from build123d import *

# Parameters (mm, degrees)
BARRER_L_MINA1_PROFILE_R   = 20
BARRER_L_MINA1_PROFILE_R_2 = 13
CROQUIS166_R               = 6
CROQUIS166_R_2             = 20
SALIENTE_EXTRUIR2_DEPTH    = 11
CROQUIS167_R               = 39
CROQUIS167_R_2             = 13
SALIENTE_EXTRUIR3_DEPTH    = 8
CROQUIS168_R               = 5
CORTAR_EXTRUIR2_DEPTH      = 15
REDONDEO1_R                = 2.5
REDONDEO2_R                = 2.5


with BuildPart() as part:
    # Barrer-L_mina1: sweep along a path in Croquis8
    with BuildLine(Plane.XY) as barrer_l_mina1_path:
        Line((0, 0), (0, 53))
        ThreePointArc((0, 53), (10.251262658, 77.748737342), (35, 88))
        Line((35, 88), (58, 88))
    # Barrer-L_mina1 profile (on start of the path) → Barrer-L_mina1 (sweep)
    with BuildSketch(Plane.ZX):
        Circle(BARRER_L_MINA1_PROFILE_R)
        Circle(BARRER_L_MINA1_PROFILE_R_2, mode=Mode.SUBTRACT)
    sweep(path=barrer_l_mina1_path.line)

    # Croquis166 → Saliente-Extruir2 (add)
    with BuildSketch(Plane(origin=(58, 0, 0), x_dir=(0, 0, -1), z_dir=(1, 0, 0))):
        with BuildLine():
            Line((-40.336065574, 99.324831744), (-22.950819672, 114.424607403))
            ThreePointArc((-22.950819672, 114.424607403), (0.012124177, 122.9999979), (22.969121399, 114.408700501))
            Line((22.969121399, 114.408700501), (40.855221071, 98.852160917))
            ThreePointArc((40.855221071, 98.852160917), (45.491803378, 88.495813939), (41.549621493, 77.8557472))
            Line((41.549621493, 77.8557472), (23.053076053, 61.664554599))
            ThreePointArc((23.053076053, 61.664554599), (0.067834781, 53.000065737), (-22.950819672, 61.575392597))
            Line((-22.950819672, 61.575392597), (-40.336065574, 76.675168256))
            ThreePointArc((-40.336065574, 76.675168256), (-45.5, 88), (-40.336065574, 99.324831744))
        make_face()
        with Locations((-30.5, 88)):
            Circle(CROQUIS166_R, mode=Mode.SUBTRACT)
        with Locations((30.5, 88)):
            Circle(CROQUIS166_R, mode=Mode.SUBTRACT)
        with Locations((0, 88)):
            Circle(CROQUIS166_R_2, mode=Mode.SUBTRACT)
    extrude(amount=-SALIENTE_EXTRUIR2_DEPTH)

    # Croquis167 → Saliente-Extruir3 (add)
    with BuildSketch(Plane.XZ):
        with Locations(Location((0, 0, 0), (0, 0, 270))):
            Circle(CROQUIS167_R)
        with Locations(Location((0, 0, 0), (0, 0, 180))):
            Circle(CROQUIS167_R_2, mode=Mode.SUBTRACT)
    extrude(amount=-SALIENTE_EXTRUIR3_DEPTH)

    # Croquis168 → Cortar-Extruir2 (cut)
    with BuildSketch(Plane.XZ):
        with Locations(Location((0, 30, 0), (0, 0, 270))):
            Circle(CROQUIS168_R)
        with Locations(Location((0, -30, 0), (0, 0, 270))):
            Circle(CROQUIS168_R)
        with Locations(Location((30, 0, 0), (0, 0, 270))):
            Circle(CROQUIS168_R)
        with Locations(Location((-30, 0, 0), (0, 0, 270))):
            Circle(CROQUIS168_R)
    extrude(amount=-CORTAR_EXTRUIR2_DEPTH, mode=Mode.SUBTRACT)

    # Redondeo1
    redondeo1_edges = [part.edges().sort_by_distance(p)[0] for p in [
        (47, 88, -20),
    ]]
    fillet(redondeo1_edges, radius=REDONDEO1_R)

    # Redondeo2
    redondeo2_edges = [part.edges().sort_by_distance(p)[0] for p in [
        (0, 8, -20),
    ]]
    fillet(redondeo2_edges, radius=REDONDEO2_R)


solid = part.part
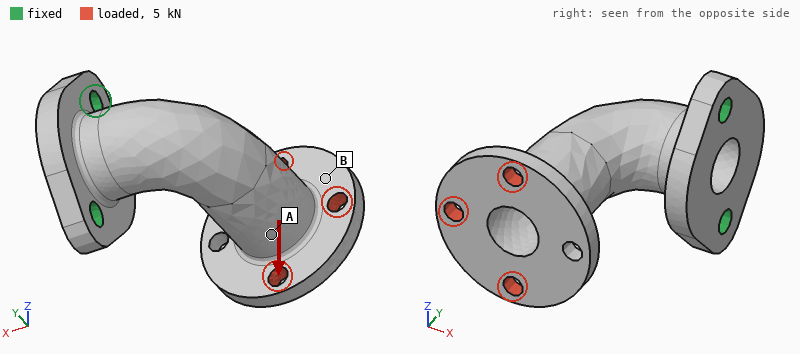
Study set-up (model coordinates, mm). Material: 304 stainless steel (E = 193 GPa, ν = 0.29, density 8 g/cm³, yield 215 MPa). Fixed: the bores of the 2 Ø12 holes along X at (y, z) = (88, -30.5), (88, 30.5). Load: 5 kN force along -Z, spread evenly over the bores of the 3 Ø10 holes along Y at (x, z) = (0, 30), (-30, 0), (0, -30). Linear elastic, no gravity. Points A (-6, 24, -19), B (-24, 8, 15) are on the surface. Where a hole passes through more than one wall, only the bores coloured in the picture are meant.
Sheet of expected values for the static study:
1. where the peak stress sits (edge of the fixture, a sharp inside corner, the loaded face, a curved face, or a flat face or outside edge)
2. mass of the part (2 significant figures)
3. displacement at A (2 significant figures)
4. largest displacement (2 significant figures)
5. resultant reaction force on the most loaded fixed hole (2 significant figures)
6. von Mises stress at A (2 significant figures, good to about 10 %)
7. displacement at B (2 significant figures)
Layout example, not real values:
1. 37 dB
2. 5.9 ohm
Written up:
1. a curved face
2. 1.2 kg
3. 0.15 mm
4. 0.24 mm
5. 9.9 kN
6. 24 MPa
7. 0.21 mm
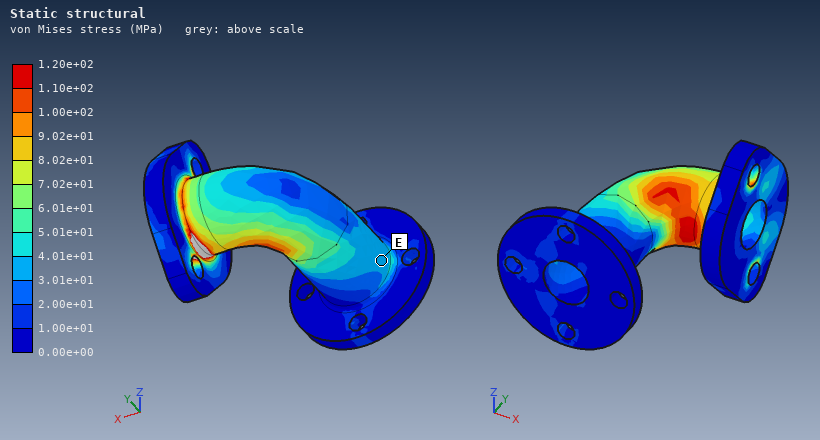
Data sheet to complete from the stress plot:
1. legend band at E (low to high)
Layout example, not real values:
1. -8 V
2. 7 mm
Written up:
1. 3.01e+01 to 4.01e+01 MPa
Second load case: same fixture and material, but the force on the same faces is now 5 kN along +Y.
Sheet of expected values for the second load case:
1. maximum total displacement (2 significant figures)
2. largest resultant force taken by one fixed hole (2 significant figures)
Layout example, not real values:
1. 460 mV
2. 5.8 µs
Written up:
1. 0.28 mm
2. 2.5 kN
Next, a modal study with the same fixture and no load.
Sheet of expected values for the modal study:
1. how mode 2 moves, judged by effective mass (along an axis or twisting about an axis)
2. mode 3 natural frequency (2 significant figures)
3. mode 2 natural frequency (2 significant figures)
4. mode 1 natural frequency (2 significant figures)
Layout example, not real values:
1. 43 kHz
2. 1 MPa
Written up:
1. along Z
2. 3200 Hz
3. 1300 Hz
4. 840 Hz
